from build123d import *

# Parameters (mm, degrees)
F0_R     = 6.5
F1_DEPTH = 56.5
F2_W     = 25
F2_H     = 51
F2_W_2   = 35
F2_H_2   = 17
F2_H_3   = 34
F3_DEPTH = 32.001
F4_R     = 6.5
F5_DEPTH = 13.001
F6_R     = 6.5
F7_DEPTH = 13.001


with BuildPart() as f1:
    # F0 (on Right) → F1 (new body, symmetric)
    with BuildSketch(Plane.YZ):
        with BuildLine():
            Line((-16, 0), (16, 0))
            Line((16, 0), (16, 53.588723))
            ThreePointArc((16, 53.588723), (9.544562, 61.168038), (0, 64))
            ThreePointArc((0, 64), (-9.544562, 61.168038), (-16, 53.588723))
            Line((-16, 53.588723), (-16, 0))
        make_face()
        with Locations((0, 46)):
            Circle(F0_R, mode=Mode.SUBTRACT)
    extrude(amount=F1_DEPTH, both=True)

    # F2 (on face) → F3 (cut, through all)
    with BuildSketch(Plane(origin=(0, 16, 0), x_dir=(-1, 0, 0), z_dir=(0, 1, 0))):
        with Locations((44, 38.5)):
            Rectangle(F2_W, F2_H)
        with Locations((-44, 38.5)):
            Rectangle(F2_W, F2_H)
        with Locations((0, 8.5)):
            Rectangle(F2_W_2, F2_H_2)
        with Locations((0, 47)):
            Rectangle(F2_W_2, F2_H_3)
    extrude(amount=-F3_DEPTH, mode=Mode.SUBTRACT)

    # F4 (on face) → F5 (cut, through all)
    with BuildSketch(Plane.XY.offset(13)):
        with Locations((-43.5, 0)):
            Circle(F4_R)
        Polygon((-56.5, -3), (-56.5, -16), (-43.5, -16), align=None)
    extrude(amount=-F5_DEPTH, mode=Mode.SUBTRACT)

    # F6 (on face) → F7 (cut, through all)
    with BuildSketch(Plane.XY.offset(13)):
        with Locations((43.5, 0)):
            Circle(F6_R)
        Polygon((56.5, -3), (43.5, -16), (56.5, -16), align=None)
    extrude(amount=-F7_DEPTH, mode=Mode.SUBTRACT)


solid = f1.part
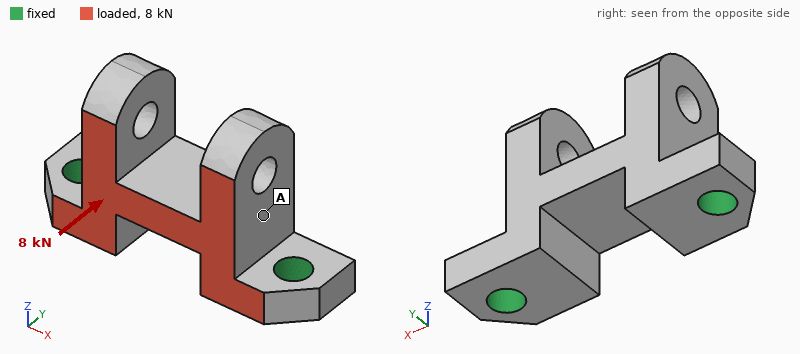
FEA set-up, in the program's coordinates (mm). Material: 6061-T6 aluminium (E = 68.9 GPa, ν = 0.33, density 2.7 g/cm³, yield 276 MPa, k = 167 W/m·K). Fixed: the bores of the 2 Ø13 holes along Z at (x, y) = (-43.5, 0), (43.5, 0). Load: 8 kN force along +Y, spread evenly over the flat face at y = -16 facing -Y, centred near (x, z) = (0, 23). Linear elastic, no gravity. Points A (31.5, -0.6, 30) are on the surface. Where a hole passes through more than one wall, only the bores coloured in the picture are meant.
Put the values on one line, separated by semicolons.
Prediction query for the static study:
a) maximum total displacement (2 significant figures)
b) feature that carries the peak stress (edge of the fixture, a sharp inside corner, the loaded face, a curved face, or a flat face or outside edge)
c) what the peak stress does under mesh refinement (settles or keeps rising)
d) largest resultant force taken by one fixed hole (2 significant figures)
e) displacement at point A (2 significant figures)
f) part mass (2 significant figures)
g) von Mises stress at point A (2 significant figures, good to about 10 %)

0.11 mm; edge of the fixture; keeps rising; 4.0 kN; 0.048 mm; 220 g; 12 MPa
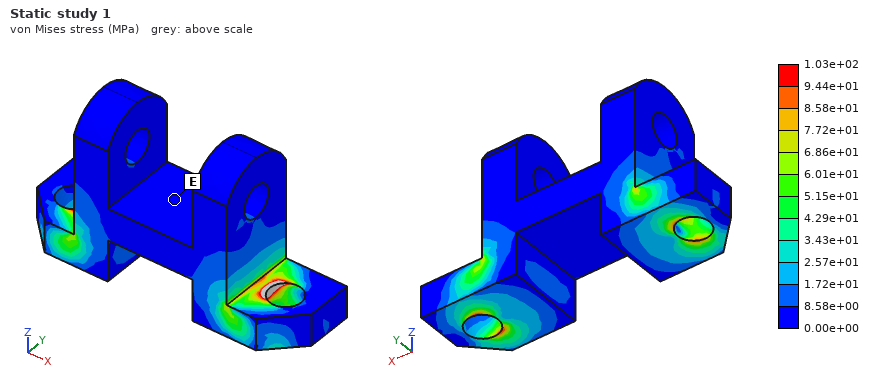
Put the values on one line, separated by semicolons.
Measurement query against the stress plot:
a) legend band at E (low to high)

0.00e+00 to 8.58e+00 MPa
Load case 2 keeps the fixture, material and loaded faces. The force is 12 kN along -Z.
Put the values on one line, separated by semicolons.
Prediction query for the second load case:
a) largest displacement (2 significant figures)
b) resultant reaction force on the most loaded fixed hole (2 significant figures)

0.13 mm; 6.7 kN
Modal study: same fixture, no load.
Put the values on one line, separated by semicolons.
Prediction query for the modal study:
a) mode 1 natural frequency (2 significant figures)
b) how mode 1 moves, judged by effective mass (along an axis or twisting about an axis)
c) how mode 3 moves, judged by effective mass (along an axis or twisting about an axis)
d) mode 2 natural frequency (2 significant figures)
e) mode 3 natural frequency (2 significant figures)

3500 Hz; along Y; along X; 5300 Hz; 5600 Hz
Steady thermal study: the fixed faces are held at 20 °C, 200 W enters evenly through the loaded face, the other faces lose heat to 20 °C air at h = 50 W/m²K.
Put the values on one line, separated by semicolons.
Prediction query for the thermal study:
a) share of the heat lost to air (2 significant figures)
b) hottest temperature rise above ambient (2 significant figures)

8.9 %; 38 K
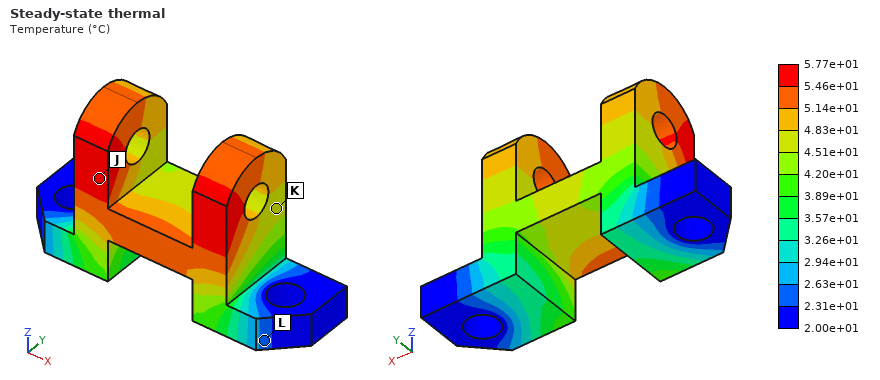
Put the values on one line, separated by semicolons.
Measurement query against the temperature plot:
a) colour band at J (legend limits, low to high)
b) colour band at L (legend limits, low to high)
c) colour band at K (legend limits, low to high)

5.46e+01 to 5.77e+01 °C; 2.31e+01 to 2.63e+01 °C; 4.51e+01 to 4.83e+01 °C
